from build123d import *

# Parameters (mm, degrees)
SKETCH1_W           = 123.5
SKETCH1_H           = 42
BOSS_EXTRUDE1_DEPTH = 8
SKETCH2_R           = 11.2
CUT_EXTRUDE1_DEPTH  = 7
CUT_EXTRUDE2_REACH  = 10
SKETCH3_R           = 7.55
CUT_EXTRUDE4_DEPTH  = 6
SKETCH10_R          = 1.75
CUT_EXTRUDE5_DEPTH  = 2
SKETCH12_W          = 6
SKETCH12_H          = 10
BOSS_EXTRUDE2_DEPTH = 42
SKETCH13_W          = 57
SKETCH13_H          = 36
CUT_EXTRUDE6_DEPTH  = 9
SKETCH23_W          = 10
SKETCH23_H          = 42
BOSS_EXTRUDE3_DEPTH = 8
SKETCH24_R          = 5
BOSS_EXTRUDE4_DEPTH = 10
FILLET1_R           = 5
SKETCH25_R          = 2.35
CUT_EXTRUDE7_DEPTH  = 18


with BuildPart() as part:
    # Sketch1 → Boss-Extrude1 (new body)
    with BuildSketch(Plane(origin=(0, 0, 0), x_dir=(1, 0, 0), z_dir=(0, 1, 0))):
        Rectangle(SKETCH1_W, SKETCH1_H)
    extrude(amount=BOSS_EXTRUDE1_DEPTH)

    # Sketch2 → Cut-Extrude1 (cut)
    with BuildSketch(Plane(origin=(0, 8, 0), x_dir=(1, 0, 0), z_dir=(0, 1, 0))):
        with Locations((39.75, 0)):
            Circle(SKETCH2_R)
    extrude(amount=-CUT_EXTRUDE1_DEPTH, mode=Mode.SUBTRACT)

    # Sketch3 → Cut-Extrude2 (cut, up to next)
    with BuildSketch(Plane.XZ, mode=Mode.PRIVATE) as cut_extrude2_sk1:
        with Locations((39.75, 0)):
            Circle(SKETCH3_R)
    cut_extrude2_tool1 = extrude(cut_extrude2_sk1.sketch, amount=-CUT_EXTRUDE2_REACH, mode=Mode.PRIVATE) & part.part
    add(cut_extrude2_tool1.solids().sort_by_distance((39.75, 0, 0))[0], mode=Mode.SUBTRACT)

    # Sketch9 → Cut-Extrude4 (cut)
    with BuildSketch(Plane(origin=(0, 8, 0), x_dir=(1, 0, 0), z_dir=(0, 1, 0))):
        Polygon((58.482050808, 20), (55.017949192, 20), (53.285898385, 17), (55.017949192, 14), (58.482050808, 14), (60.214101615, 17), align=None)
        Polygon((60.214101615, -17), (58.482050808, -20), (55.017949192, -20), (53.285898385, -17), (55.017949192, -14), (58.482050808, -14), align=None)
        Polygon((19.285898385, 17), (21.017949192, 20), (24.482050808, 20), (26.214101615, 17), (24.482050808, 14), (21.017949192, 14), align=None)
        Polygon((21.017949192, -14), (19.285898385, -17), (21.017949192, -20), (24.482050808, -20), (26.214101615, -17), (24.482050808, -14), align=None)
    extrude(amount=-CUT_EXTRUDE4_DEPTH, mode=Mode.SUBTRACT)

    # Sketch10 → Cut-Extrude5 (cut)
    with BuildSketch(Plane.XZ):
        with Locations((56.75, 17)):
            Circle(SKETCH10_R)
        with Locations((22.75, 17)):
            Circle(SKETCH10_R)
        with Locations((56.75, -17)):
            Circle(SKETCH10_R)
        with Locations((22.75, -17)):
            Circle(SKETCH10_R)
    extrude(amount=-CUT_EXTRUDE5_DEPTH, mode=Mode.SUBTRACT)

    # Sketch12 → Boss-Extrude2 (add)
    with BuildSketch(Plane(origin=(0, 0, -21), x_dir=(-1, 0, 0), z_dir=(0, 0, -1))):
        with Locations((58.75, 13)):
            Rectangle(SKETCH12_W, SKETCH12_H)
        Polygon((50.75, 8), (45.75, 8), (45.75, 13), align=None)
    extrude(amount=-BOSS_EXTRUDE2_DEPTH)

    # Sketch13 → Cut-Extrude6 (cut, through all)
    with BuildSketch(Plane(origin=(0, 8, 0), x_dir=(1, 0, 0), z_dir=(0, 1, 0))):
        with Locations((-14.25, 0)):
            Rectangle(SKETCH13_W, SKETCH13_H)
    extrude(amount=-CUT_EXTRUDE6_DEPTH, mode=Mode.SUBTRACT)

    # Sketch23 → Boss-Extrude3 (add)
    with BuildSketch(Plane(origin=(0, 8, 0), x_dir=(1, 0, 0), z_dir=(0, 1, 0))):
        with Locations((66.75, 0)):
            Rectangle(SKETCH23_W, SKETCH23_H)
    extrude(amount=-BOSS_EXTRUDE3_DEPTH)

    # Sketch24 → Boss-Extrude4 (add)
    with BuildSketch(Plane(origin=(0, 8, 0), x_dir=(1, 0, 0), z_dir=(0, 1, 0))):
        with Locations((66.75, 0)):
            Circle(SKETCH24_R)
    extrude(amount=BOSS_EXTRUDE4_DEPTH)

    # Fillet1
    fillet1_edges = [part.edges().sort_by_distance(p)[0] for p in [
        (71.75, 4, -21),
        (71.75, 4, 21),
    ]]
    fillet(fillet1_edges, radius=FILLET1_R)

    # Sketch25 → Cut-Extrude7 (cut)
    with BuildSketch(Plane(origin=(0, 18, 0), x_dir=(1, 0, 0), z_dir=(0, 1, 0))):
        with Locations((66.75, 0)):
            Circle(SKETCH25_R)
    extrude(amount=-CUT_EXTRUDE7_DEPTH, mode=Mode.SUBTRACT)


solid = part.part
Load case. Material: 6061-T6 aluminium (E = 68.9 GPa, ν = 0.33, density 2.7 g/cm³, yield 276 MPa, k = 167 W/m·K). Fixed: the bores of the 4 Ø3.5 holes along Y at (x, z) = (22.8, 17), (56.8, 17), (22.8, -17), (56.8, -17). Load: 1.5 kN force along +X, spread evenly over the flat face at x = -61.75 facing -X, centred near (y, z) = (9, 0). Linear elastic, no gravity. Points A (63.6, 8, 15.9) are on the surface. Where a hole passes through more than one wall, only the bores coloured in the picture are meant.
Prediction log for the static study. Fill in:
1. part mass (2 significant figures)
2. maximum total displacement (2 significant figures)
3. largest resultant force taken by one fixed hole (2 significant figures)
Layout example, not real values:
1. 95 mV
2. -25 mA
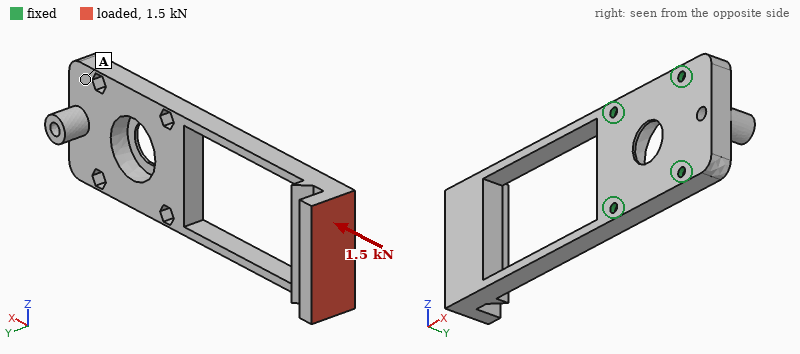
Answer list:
1. 76 g
2. 1.6 mm
3. 480 N
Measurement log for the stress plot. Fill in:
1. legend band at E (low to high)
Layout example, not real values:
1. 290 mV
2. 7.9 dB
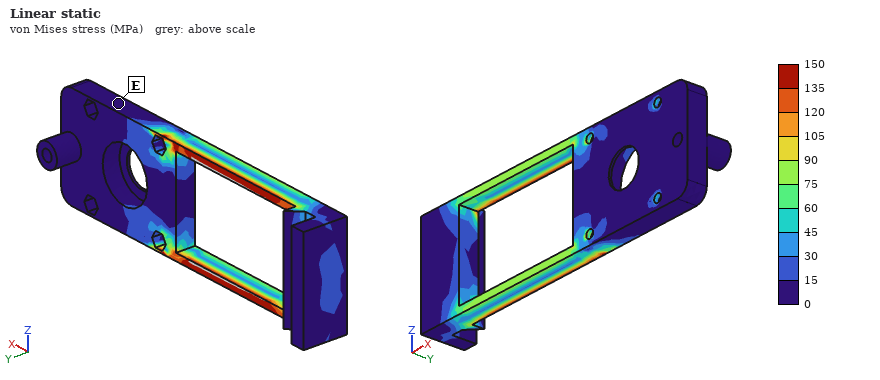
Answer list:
1. 0 to 15 MPa
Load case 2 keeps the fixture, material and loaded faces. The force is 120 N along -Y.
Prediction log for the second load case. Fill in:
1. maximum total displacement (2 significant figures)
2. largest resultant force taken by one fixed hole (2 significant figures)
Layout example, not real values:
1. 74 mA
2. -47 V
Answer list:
1. 1.4 mm
2. 400 N
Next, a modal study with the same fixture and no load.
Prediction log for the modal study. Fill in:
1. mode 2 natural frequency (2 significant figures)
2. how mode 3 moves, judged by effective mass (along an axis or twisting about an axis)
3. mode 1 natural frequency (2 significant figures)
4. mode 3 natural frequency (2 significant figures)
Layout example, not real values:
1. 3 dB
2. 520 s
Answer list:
1. 350 Hz
2. twisting about X
3. 340 Hz
4. 1200 Hz
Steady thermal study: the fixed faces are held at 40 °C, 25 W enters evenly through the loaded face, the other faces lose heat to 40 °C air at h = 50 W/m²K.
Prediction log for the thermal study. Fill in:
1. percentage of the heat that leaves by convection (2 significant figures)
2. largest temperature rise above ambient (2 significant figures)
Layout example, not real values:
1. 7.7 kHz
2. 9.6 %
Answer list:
1. 69 %
2. 85 K
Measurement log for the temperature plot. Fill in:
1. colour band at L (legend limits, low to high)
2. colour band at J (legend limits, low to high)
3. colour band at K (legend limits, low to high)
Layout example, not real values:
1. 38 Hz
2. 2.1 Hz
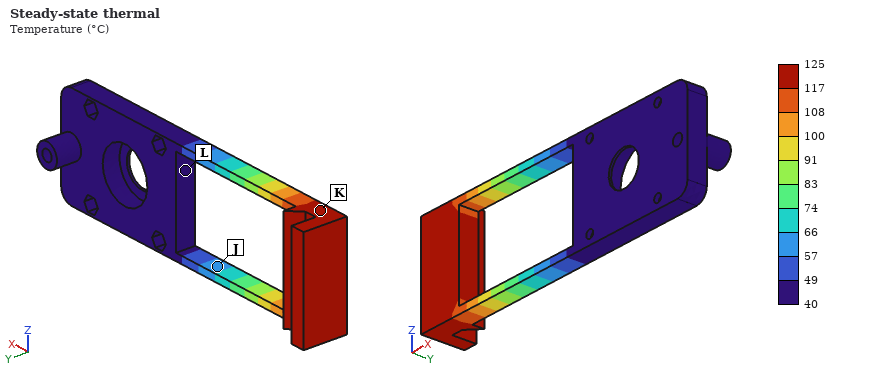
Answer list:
1. 40 to 49 °C
2. 57 to 66 °C
3. 117 to 125 °C
